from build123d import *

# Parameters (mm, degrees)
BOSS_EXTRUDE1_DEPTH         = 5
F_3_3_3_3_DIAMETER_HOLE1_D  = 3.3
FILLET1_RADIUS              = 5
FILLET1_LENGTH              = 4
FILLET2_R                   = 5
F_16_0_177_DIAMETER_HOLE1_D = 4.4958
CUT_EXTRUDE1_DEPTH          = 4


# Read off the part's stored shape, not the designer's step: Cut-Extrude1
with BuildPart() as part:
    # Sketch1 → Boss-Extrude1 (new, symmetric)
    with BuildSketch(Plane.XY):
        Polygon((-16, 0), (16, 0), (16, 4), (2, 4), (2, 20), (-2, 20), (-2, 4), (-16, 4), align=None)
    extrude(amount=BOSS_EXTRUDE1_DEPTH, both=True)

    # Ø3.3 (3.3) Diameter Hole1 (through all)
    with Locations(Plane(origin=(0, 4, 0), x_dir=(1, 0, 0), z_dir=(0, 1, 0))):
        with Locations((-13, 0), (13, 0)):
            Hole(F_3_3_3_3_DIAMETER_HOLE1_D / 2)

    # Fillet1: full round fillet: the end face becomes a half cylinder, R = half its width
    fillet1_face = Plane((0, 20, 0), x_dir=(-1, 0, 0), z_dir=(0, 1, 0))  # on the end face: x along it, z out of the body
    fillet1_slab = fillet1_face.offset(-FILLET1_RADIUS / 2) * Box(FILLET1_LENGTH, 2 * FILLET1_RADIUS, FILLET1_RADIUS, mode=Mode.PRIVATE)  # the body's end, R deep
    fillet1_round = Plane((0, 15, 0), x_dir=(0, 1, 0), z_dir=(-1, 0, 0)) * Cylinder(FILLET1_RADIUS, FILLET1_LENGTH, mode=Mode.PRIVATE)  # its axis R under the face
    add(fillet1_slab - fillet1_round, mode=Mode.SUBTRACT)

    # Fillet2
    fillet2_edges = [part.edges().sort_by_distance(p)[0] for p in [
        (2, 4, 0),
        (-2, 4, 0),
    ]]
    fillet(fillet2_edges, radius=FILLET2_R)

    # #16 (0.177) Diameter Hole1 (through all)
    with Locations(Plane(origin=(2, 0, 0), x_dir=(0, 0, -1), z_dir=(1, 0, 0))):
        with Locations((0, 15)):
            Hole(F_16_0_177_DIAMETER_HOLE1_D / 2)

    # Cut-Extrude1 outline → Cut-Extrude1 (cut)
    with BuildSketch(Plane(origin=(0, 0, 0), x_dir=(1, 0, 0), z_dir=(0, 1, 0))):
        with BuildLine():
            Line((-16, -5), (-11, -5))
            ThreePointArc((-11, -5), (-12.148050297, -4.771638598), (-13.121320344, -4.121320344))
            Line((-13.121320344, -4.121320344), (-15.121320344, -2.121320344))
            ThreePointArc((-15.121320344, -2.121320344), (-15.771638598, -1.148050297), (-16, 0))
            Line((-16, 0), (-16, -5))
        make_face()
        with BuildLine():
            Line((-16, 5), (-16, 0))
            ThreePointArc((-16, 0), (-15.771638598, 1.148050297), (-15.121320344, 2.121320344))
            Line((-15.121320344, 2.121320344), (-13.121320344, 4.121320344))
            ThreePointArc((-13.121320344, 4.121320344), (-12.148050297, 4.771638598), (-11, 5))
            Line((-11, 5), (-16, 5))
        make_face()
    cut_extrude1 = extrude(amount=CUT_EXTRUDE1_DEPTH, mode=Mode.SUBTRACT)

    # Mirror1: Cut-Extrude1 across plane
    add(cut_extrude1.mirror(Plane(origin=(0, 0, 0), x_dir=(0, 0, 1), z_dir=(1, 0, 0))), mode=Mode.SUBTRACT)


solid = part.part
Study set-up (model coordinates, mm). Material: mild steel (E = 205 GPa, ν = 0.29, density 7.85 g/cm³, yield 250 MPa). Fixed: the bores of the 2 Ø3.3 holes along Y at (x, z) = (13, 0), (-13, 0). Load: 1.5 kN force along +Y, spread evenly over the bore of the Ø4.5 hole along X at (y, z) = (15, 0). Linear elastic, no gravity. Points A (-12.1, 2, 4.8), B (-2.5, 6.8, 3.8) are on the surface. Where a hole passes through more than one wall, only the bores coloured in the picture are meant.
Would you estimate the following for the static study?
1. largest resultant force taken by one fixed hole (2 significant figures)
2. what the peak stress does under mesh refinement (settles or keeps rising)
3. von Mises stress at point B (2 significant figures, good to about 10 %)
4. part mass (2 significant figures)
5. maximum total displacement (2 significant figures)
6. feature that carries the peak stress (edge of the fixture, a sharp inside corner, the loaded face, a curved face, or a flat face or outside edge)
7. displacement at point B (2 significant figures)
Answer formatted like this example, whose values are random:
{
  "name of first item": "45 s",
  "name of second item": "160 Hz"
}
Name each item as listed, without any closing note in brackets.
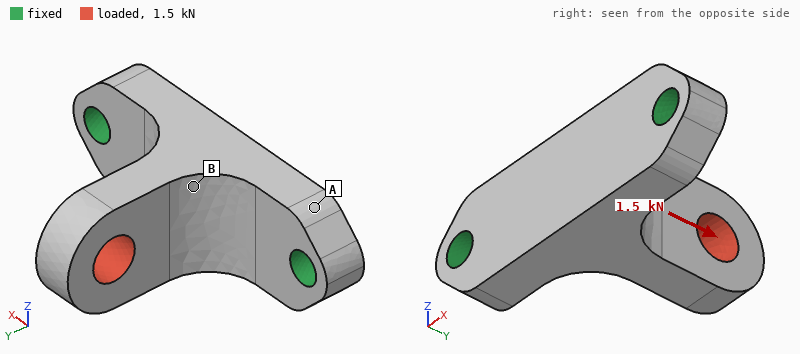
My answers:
{
  "largest resultant force taken by one fixed hole": "820 N",
  "what the peak stress does under mesh refinement": "keeps rising",
  "von Mises stress at point B": "54 MPa",
  "part mass": "14 g",
  "maximum total displacement": "11 µm",
  "feature that carries the peak stress": "edge of the fixture",
  "displacement at point B": "8.1 µm"
}
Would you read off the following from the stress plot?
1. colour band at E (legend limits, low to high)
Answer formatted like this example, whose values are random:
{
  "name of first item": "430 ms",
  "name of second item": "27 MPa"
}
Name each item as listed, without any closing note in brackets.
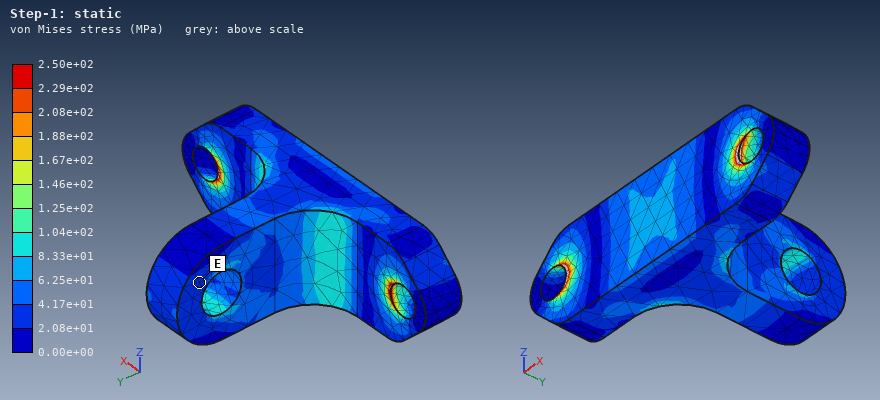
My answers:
{
  "colour band at E": "2.08e+01 to 4.17e+01 MPa"
}
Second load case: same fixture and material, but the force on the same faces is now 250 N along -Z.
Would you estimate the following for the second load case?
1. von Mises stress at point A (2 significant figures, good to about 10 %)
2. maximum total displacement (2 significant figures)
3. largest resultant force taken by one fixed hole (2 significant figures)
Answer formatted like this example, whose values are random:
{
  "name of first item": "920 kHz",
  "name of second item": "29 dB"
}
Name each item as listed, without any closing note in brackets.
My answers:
{
  "von Mises stress at point A": "25 MPa",
  "maximum total displacement": "23 µm",
  "largest resultant force taken by one fixed hole": "130 N"
}
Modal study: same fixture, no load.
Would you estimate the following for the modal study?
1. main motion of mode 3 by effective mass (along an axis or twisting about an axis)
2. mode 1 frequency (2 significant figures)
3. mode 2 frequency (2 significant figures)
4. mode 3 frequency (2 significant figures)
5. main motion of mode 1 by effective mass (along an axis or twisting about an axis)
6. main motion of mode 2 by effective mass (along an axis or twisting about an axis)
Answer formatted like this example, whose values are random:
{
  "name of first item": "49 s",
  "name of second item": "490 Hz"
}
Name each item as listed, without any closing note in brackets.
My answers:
{
  "main motion of mode 3 by effective mass": "along Y",
  "mode 1 frequency": "11 kHz",
  "mode 2 frequency": "17 kHz",
  "mode 3 frequency": "23 kHz",
  "main motion of mode 1 by effective mass": "along Z",
  "main motion of mode 2 by effective mass": "along X"
}
